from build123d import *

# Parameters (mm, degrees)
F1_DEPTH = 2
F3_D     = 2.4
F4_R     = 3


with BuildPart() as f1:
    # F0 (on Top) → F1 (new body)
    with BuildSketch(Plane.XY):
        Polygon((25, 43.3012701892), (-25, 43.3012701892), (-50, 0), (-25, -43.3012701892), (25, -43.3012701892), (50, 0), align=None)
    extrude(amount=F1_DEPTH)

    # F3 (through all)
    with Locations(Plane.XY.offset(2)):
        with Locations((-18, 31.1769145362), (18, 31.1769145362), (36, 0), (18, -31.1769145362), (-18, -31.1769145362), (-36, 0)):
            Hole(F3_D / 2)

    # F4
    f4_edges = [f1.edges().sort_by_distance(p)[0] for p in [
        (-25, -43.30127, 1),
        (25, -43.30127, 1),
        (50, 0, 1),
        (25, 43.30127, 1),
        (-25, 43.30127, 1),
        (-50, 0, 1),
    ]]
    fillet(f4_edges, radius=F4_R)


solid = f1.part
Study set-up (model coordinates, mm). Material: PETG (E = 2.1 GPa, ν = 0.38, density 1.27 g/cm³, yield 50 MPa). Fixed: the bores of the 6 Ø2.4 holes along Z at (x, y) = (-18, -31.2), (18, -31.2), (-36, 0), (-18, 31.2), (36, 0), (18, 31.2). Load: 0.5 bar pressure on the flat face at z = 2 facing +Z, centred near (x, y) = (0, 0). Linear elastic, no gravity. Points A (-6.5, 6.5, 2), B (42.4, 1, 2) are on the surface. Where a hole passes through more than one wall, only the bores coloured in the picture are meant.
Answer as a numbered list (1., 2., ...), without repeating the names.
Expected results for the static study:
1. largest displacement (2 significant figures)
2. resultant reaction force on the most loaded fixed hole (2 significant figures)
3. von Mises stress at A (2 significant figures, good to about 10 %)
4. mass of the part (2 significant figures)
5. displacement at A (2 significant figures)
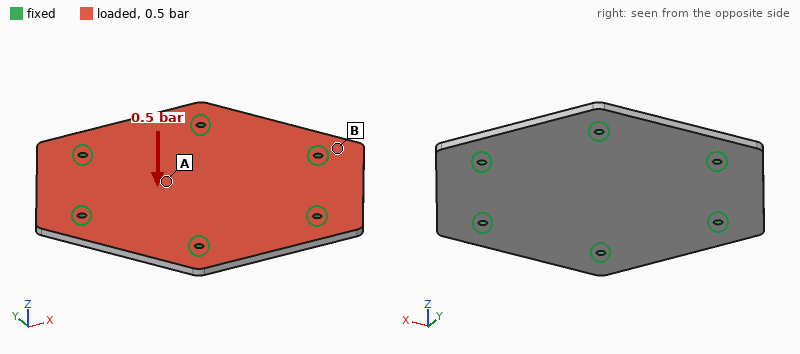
1. 1.1 mm
2. 54 N
3. 8.2 MPa
4. 16 g
5. 0.97 mm
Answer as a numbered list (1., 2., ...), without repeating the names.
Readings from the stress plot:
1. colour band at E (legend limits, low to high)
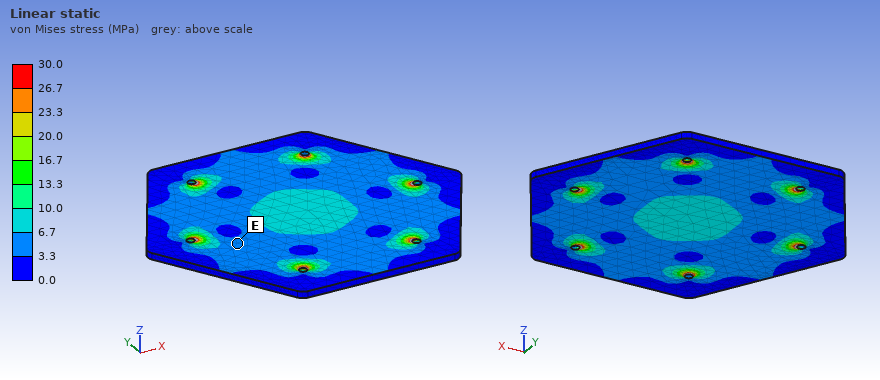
1. 3.3 to 6.7 MPa
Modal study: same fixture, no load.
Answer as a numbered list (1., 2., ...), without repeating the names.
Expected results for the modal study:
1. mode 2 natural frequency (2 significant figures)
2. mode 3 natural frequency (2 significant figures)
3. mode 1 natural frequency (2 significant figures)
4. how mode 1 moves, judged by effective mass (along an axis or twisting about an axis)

1. 1500 Hz
2. 1600 Hz
3. 820 Hz
4. along Z
